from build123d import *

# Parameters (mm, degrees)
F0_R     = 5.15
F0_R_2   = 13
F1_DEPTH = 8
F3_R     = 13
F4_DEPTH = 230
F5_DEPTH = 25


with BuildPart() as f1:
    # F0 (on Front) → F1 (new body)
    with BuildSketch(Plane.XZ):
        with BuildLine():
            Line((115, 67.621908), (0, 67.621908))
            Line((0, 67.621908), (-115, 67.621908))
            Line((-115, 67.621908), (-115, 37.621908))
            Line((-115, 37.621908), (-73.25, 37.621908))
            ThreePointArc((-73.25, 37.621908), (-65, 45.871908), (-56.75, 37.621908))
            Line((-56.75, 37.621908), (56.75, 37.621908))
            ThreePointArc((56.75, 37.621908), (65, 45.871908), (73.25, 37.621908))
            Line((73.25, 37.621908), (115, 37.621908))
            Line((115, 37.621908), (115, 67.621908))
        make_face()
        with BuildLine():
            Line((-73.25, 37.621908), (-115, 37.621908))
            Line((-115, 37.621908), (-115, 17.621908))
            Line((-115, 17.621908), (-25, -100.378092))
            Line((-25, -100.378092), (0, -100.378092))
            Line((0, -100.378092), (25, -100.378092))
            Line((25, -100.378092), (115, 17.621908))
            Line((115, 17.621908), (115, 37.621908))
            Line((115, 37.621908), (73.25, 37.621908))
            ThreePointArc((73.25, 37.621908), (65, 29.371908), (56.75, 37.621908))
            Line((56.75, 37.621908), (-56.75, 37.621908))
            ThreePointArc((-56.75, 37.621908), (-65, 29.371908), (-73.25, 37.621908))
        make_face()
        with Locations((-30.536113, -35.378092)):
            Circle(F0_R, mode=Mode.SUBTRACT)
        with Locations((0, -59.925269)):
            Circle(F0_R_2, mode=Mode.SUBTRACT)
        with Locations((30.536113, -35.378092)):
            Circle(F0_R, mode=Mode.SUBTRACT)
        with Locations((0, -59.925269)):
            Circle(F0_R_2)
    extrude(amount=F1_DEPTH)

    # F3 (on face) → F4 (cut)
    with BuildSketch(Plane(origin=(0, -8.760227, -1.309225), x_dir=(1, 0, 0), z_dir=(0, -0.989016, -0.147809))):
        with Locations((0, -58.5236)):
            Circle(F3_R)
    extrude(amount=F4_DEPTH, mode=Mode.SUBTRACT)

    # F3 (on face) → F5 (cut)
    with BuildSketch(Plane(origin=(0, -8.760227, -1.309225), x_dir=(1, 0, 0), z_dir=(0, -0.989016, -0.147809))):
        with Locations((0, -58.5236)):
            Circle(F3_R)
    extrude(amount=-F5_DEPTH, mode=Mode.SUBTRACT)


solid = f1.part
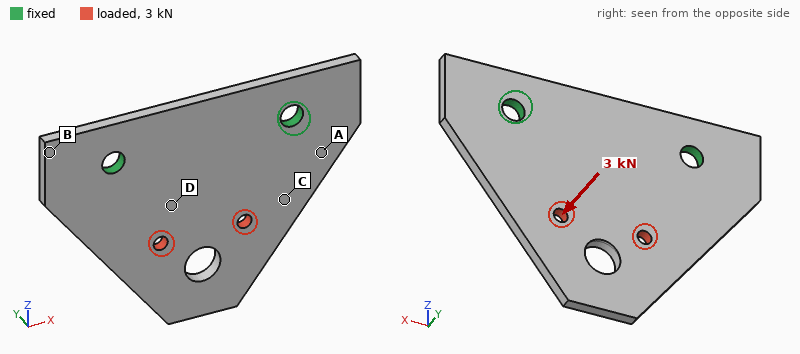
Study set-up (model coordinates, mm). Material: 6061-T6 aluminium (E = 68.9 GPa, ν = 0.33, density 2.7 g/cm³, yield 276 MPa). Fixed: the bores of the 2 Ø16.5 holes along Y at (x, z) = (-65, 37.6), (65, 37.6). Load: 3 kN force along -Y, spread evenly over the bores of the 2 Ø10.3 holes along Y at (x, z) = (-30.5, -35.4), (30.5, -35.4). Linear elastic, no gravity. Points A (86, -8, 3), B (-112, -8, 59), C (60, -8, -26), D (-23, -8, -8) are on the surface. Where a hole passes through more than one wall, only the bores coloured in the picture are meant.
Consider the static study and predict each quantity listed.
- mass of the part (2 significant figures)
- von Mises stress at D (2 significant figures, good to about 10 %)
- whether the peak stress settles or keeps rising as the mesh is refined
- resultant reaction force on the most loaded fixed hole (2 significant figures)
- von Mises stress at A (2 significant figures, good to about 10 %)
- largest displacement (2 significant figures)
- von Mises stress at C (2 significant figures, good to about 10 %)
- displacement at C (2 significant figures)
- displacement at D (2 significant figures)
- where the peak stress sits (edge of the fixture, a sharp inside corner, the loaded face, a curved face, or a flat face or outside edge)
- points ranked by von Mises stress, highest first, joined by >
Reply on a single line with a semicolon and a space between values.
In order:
580 g; 44 MPa; keeps rising; 1.5 kN; 67 MPa; 1.9 mm; 31 MPa; 0.56 mm; 0.45 mm; edge of the fixture; A > D > C > B
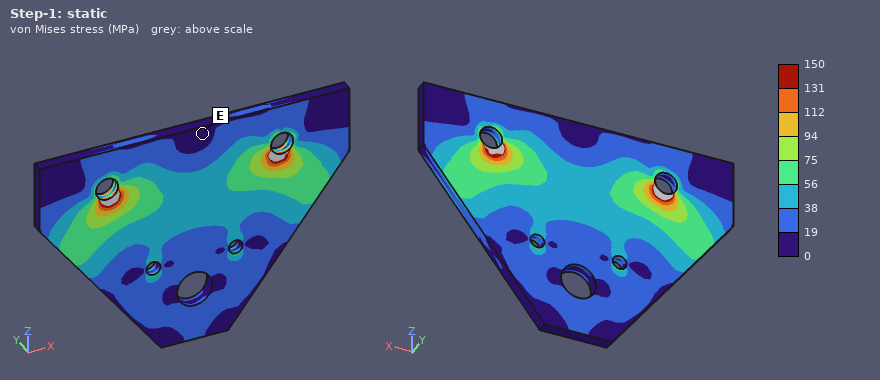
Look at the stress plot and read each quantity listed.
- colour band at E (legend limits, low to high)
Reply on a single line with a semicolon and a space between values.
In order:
0 to 19 MPa
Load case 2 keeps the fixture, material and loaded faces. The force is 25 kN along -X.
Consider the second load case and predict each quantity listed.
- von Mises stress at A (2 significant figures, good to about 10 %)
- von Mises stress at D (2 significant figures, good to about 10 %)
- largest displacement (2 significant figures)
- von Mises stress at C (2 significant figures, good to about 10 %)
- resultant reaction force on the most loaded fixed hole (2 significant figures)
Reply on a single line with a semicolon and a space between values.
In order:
14 MPa; 39 MPa; 84 µm; 23 MPa; 18 kN
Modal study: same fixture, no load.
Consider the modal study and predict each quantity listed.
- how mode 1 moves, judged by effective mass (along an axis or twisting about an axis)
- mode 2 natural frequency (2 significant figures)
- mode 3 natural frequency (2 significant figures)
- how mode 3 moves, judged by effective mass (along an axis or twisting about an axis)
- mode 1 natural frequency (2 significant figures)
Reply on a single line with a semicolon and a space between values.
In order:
along Y; 1400 Hz; 2000 Hz; along Y; 480 Hz
